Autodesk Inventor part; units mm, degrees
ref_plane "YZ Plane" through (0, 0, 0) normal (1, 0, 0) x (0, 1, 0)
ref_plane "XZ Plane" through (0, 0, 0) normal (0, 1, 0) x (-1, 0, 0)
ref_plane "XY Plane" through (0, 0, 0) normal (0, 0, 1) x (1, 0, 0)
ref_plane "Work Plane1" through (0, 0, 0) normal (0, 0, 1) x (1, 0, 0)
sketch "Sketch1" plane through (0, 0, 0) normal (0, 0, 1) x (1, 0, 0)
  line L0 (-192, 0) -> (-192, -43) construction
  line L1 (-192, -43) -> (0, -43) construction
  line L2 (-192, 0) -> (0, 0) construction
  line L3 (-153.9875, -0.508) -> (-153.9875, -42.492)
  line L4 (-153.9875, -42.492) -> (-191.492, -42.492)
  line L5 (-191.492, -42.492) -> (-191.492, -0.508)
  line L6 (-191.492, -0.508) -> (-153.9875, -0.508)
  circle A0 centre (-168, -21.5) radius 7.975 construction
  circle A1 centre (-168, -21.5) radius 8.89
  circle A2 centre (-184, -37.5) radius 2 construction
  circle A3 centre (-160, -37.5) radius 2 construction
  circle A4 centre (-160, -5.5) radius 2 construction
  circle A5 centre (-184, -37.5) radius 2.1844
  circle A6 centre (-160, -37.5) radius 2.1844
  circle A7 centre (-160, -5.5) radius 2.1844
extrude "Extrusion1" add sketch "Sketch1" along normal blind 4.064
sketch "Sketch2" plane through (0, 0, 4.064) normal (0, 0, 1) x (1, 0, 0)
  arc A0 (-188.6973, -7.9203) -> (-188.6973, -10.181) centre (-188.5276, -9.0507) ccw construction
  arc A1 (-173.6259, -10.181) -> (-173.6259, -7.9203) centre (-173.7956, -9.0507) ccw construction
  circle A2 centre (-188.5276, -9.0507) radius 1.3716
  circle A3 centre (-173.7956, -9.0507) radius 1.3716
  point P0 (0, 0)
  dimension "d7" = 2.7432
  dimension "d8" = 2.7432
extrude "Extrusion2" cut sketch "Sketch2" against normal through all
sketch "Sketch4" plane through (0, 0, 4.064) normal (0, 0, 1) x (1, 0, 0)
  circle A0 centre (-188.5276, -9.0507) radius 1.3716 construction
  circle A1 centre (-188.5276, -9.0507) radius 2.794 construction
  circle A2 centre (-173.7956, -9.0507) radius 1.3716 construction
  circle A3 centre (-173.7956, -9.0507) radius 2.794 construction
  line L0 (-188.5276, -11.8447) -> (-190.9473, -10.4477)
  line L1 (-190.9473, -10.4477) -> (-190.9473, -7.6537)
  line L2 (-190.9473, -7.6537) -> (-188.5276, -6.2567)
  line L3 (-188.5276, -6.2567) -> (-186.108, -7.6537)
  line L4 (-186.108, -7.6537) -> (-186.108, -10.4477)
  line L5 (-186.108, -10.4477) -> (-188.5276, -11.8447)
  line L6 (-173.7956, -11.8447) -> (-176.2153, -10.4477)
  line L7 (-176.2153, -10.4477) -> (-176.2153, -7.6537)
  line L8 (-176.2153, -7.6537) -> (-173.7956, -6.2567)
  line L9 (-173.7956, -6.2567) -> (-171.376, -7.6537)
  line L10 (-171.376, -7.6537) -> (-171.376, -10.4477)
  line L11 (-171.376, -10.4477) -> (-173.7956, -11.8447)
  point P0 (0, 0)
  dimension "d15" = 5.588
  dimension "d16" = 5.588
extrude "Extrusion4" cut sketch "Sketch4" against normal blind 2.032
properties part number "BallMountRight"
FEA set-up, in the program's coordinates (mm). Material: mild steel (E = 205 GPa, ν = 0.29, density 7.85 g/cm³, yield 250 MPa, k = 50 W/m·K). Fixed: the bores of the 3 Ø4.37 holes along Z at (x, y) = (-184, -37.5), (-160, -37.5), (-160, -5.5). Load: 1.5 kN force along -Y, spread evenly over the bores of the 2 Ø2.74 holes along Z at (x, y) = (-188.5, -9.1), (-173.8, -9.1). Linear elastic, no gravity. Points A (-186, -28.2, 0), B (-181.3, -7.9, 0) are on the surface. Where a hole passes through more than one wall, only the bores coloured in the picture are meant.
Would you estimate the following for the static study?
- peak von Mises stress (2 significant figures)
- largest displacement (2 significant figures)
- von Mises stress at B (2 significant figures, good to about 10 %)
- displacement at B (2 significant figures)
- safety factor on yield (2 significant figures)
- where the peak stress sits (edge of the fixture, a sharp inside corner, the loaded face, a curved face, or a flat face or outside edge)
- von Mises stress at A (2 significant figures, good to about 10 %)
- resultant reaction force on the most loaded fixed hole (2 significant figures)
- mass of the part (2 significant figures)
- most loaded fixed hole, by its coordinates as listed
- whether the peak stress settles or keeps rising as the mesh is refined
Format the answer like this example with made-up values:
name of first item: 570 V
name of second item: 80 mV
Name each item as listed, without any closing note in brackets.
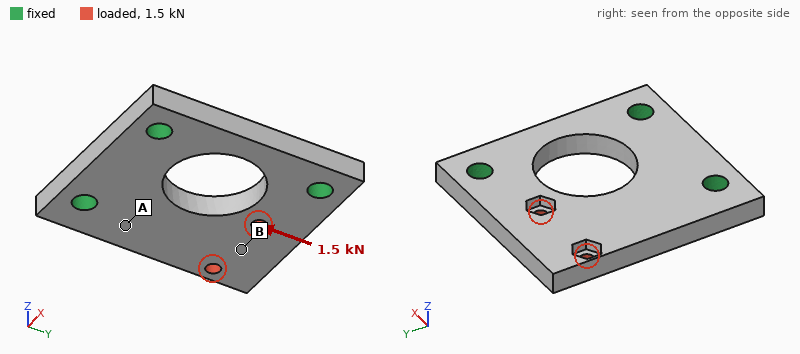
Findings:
peak von Mises stress: 100 MPa
largest displacement: 13 µm
von Mises stress at B: 12 MPa
displacement at B: 5.5 µm
safety factor on yield: 2.4
where the peak stress sits: the loaded face
von Mises stress at A: 26 MPa
resultant reaction force on the most loaded fixed hole: 1.0 kN
mass of the part: 40 g
most loaded fixed hole, by its coordinates as listed: (-184, -37.5)
whether the peak stress settles or keeps rising as the mesh is refined: settles
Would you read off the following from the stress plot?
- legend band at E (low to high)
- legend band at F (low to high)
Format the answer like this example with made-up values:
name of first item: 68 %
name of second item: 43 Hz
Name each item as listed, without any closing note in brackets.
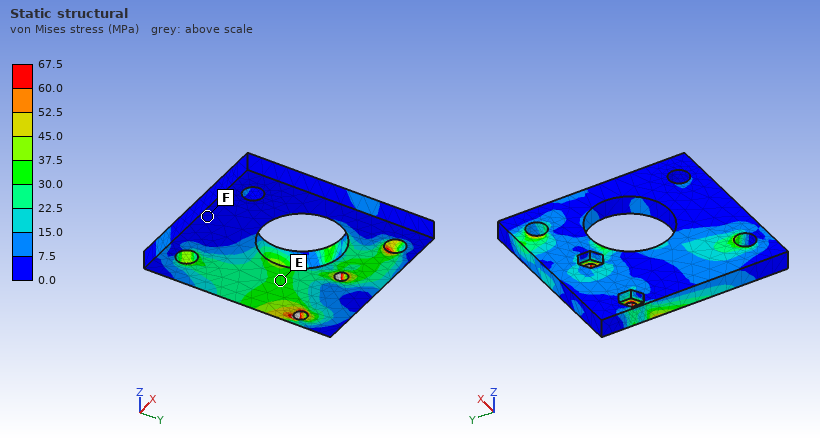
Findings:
legend band at E: 30.0 to 37.5 MPa
legend band at F: 0.0 to 7.5 MPa
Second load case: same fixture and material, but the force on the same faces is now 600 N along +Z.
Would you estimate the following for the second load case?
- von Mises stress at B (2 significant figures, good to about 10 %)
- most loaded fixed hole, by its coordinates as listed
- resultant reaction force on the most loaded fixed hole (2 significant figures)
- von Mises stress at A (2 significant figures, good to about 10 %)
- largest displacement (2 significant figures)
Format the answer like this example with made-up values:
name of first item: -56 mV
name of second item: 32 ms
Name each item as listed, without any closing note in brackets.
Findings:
von Mises stress at B: 53 MPa
most loaded fixed hole, by its coordinates as listed: (-160, -5.5)
resultant reaction force on the most loaded fixed hole: 400 N
von Mises stress at A: 64 MPa
largest displacement: 77 µm
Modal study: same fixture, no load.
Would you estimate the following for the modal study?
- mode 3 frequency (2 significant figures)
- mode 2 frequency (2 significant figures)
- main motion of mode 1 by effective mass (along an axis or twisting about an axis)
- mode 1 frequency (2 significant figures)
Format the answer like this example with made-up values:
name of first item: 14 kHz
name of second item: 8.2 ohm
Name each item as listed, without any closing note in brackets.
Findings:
mode 3 frequency: 20 kHz
mode 2 frequency: 16 kHz
main motion of mode 1 by effective mass: along Z
mode 1 frequency: 5500 Hz
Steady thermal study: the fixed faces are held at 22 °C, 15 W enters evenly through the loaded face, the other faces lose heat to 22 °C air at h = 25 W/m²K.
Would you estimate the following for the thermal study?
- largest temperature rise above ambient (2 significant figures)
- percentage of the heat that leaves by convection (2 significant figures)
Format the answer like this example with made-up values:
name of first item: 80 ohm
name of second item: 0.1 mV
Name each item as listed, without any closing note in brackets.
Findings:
largest temperature rise above ambient: 71 K
percentage of the heat that leaves by convection: 10 %
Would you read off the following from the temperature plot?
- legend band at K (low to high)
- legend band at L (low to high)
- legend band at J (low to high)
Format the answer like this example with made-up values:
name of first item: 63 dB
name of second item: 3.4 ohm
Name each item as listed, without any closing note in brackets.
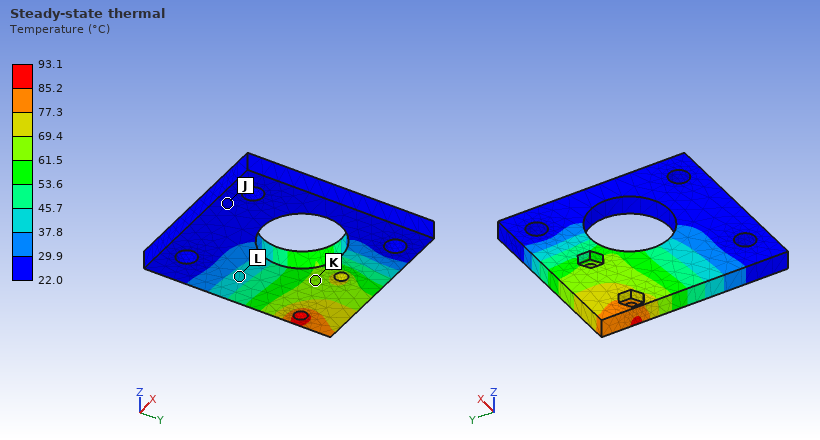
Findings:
legend band at K: 61.5 to 69.4 °C
legend band at L: 37.8 to 45.7 °C
legend band at J: 22.0 to 29.9 °C
